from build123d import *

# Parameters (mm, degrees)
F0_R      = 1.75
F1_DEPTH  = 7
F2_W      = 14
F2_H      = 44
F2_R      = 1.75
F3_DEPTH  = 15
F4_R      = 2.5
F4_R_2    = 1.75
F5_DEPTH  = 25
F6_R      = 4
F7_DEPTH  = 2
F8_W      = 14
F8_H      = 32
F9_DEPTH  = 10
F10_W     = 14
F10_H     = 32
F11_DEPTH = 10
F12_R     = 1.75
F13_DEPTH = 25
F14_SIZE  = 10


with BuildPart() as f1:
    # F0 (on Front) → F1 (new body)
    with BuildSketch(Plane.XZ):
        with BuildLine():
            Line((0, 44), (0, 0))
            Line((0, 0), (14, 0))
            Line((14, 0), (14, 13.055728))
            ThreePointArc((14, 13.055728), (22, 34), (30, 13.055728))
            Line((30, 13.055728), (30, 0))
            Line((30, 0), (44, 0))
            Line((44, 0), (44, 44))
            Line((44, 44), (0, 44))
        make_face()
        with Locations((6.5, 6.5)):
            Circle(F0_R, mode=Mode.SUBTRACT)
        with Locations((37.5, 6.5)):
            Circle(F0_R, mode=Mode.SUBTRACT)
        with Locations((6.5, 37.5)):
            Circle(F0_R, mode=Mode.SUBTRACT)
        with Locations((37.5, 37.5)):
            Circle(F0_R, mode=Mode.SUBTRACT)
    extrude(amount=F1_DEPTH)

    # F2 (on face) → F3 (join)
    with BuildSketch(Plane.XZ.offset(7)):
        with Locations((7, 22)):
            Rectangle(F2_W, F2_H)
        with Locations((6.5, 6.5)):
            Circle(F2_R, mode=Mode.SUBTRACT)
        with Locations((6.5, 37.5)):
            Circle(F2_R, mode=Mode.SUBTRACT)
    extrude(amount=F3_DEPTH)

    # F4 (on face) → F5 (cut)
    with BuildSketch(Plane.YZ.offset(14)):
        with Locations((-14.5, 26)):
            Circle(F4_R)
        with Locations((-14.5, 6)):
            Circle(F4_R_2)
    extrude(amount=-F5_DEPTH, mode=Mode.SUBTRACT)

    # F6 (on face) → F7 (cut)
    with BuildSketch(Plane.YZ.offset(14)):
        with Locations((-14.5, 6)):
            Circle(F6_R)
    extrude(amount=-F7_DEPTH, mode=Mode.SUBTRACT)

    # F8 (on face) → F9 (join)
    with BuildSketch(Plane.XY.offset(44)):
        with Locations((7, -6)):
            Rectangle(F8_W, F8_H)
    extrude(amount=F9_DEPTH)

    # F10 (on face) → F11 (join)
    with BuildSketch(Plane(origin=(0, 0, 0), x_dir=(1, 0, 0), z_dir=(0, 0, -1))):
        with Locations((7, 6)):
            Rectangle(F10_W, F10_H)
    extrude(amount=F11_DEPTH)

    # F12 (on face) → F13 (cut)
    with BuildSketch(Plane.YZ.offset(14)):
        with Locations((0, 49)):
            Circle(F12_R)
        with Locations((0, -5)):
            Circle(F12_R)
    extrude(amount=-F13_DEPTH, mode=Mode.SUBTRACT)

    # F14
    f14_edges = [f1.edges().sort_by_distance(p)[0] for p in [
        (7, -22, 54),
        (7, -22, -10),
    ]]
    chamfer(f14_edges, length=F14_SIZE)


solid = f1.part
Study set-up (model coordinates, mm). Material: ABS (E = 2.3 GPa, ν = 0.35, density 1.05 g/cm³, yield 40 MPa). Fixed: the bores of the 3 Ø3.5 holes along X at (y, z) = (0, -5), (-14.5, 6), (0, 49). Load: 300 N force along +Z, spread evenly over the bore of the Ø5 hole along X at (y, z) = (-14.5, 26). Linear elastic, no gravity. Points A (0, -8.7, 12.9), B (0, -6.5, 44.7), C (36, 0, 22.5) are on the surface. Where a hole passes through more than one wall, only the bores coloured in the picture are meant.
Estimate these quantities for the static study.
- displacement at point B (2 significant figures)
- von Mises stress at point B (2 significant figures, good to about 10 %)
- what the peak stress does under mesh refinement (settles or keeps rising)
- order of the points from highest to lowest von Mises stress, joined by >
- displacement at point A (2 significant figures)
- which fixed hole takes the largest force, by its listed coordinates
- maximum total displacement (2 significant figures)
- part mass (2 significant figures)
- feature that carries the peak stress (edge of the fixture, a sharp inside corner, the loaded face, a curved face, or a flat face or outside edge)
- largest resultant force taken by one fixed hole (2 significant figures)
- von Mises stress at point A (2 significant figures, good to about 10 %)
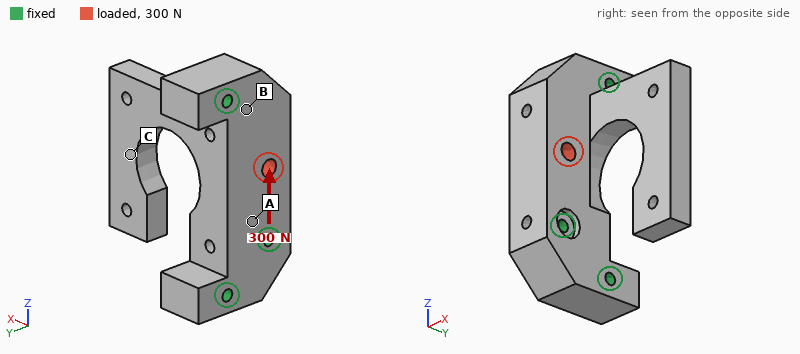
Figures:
4.8 µm
0.51 MPa
keeps rising
A > B > C
4.5 µm
(-14.5, 6)
16 µm
26 g
edge of the fixture
170 N
0.72 MPa
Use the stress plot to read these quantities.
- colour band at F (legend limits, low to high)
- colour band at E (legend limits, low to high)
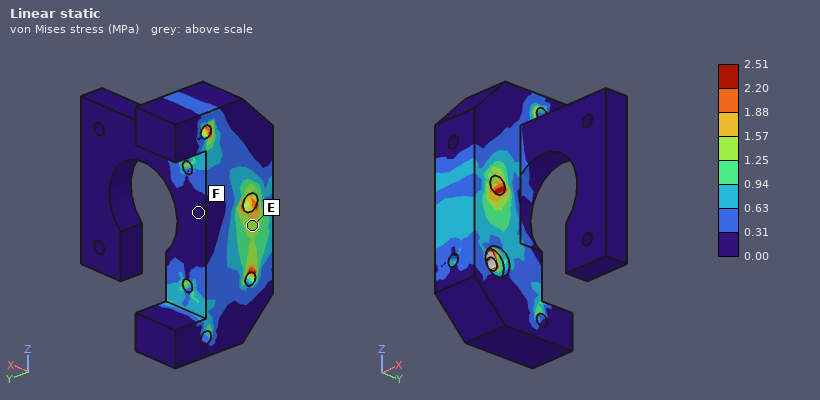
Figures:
0.00 to 0.31 MPa
1.25 to 1.57 MPa
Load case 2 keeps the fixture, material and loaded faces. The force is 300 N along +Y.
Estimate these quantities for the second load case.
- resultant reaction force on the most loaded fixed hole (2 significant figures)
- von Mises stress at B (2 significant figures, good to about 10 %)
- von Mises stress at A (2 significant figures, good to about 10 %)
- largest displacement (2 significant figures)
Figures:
160 N
1.2 MPa
1.5 MPa
62 µm
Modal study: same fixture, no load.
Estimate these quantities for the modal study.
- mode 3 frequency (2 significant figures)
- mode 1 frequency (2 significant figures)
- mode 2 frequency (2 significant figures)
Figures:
1300 Hz
490 Hz
740 Hz
